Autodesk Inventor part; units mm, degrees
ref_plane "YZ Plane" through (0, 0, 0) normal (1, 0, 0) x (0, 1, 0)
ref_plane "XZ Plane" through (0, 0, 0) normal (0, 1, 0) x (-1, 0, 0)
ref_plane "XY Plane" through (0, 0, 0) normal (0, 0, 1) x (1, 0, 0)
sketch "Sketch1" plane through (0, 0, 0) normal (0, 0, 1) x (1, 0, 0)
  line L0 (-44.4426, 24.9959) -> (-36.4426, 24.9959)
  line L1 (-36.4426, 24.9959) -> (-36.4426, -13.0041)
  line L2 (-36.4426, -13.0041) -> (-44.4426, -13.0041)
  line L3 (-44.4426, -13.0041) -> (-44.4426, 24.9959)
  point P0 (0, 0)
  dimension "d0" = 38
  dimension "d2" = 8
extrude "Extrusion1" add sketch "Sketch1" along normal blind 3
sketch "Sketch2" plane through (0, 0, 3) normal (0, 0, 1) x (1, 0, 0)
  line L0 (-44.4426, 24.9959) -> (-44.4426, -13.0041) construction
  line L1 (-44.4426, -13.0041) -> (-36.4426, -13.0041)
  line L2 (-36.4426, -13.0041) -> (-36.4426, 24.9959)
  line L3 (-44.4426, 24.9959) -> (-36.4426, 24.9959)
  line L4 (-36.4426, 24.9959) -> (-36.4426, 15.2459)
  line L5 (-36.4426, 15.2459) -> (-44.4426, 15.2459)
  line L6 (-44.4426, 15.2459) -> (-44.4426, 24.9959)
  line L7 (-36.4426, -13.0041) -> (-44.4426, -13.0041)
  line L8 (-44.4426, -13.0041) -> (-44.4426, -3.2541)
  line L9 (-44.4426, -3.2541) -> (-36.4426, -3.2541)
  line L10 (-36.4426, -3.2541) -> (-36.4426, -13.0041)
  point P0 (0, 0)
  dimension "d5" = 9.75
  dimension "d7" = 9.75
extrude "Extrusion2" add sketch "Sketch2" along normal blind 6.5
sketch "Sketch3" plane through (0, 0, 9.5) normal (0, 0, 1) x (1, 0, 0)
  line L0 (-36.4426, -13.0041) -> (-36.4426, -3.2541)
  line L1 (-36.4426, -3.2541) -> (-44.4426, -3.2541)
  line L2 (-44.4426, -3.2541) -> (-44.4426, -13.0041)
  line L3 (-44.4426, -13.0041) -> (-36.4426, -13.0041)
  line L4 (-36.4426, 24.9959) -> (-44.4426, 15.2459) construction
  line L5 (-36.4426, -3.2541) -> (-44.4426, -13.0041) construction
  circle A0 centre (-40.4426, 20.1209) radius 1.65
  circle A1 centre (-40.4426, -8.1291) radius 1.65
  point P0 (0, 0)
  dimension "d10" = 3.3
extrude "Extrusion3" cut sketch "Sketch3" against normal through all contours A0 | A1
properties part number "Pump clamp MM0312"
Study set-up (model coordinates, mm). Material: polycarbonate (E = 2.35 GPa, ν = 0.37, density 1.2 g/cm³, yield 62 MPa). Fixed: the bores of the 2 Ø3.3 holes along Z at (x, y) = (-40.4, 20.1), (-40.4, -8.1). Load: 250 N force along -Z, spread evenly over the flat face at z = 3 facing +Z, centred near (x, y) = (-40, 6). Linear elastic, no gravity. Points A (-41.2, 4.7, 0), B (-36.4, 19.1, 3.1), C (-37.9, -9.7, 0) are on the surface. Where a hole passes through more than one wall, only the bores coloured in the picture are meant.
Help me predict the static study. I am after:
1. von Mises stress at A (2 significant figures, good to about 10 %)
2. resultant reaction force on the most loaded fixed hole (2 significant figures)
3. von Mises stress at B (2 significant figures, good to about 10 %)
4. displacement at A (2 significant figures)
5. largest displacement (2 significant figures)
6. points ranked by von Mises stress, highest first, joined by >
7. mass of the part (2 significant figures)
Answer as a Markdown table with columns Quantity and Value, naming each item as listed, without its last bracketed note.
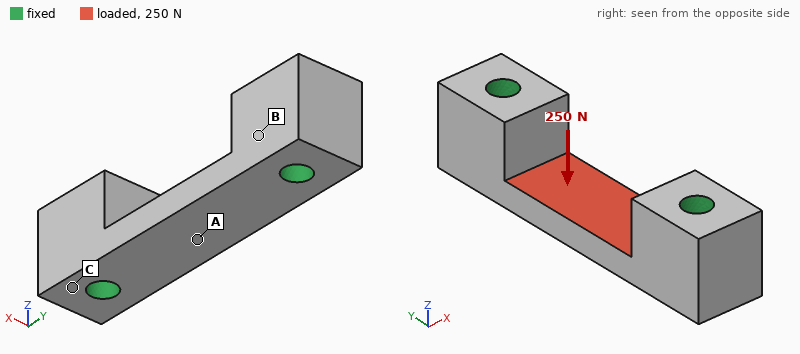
| Quantity | Value |
|---|---|
| von Mises stress at A | 21 MPa |
| resultant reaction force on the most loaded fixed hole | 130 N |
| von Mises stress at B | 4.1 MPa |
| displacement at A | 0.20 mm |
| largest displacement | 0.22 mm |
| points ranked by von Mises stress, highest first, joined by > | A > B > C |
| mass of the part | 2.1 g |
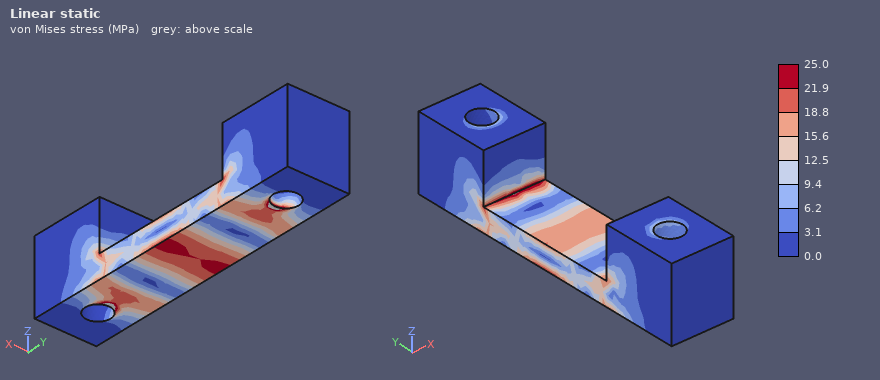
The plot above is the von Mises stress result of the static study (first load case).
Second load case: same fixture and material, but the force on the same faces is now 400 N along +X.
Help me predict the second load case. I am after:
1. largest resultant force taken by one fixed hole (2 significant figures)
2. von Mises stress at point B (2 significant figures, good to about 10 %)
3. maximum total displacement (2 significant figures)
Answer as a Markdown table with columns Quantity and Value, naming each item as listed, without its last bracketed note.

| Quantity | Value |
|---|---|
| largest resultant force taken by one fixed hole | 200 N |
| von Mises stress at point B | 11 MPa |
| maximum total displacement | 0.25 mm |
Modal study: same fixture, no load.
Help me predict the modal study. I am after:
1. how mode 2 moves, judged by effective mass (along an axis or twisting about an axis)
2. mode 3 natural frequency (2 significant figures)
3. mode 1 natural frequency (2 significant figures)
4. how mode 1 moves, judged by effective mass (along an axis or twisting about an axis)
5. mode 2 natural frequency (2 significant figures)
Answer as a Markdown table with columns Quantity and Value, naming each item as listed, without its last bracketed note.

| Quantity | Value |
|---|---|
| how mode 2 moves, judged by effective mass | along X |
| mode 3 natural frequency | 14 kHz |
| mode 1 natural frequency | 8300 Hz |
| how mode 1 moves, judged by effective mass | along Z |
| mode 2 natural frequency | 11 kHz |
